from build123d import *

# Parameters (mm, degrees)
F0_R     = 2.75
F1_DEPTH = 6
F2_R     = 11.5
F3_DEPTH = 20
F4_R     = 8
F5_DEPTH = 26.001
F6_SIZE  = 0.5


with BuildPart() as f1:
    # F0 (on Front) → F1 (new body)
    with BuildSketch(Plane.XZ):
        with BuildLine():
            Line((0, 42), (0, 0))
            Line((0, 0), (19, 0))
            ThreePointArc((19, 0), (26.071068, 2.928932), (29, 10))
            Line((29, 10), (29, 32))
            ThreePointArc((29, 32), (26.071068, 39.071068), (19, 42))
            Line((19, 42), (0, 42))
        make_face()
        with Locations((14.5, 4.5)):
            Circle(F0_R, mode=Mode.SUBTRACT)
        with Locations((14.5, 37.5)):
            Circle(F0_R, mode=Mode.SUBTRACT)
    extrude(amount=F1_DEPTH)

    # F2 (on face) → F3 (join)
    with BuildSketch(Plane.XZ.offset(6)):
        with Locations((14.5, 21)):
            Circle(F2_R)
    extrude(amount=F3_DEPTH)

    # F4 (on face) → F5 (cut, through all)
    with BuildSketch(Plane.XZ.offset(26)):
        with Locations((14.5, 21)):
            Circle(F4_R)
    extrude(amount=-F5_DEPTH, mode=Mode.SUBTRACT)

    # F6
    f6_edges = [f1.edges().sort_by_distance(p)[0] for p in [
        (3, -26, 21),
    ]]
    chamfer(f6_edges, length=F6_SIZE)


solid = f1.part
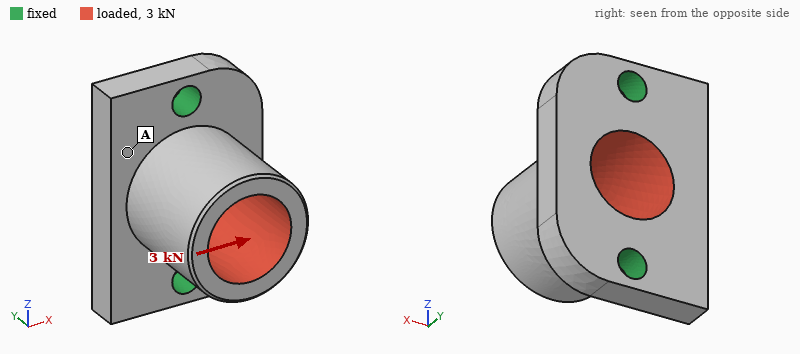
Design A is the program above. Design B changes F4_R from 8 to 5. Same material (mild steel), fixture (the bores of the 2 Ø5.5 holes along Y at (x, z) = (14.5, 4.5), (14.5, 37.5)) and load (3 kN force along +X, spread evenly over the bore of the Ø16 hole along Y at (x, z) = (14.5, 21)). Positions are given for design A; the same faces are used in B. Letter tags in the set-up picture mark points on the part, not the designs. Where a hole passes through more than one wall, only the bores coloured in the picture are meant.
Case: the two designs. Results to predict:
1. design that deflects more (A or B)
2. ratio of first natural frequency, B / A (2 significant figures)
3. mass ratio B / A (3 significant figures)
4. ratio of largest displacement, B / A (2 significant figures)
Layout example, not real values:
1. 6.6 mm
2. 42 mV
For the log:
1. A
2. 0.88
3. 1.32
4. 0.89
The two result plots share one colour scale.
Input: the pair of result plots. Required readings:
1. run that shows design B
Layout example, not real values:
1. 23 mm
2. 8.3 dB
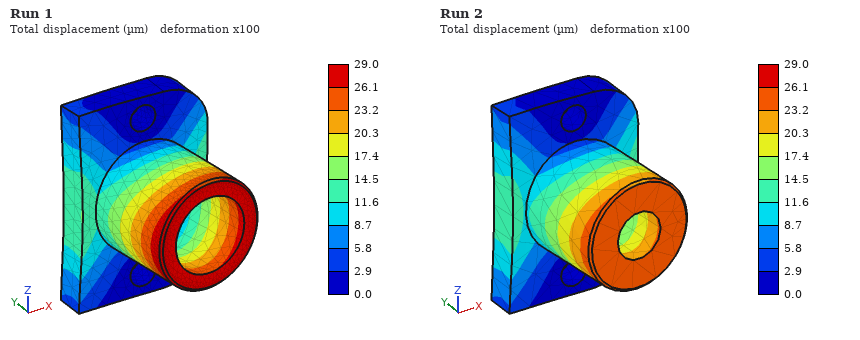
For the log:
1. Run 2
